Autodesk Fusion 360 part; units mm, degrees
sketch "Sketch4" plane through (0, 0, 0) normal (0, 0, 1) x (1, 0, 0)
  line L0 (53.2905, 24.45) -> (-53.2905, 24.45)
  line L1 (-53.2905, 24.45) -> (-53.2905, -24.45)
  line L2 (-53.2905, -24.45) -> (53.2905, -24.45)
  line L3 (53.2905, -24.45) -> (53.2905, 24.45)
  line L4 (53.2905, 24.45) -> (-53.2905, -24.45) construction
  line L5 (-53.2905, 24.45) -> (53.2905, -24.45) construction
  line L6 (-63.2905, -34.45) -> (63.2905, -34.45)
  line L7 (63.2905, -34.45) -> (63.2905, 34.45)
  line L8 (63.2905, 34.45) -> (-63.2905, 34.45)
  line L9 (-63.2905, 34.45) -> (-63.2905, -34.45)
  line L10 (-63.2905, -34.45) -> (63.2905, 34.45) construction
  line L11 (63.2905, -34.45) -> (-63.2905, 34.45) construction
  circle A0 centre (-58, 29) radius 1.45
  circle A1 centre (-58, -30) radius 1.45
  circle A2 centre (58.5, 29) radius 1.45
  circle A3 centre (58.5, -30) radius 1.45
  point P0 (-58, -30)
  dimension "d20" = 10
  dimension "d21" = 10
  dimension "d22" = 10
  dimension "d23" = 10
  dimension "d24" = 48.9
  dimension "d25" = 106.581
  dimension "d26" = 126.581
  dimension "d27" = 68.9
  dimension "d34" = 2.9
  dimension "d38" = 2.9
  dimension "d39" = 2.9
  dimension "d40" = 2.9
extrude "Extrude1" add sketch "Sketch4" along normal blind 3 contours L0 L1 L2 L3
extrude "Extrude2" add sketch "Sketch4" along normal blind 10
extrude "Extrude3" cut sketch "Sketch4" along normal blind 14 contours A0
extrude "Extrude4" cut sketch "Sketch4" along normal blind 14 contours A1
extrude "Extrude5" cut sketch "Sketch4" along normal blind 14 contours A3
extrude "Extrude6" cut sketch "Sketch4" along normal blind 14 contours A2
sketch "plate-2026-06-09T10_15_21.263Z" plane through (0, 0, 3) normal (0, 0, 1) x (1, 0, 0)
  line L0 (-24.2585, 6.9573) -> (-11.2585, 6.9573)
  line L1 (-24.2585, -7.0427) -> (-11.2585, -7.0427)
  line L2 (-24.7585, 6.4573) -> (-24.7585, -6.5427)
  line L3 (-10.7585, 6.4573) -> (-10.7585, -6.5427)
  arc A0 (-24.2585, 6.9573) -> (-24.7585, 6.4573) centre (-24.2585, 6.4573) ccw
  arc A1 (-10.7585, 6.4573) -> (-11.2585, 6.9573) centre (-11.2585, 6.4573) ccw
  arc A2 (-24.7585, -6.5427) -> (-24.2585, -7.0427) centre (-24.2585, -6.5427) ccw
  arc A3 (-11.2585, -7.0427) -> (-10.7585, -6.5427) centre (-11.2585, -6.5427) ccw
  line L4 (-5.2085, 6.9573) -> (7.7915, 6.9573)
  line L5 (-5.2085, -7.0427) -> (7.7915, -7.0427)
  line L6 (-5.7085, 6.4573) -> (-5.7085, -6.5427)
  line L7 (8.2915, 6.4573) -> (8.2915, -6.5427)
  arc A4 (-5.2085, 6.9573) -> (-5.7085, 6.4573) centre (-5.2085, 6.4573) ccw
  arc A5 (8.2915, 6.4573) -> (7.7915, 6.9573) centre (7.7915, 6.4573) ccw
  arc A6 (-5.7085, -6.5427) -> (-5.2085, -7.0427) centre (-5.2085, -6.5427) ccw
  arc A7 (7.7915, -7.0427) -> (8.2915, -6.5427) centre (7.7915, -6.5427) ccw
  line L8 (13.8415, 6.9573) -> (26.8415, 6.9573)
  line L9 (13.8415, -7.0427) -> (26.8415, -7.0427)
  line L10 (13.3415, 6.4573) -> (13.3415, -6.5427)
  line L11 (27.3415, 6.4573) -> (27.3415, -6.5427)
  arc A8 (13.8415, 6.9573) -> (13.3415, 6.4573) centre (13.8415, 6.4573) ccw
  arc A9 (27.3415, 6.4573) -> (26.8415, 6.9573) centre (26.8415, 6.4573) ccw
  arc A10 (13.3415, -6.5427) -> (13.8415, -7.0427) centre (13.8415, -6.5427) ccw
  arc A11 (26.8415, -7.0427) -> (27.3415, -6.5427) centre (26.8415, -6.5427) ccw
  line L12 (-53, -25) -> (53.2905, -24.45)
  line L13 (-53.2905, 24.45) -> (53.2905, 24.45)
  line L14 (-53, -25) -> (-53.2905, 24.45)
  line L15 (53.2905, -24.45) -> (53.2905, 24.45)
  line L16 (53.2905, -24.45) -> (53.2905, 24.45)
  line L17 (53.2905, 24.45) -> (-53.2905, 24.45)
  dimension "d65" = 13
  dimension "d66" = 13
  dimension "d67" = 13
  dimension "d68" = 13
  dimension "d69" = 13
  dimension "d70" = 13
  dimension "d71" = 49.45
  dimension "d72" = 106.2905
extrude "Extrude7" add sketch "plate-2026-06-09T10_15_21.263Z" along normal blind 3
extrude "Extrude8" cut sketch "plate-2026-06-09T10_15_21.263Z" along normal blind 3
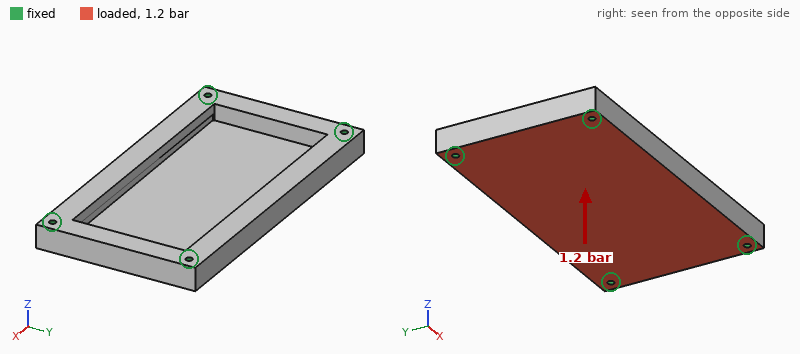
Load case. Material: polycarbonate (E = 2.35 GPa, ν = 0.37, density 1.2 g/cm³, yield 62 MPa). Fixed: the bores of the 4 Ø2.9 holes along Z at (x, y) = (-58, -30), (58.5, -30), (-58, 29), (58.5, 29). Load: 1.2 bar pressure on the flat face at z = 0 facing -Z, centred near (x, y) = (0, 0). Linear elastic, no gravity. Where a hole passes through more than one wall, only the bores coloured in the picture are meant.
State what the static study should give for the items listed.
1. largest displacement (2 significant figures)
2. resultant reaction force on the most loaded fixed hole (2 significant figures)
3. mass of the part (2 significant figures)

1.5 mm
310 N
60 g
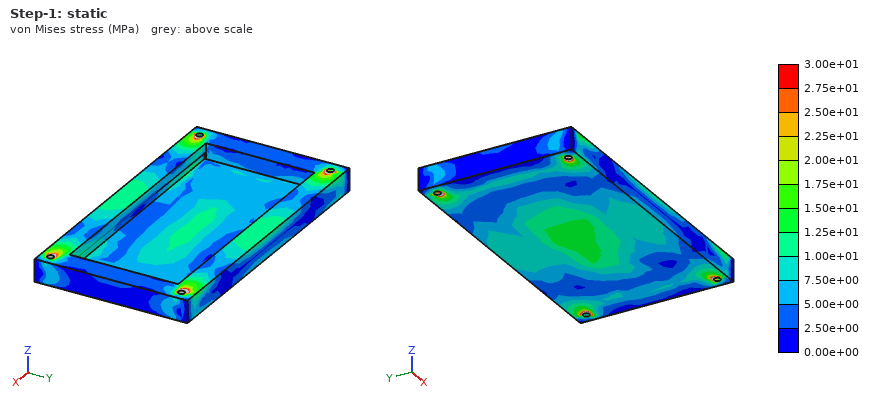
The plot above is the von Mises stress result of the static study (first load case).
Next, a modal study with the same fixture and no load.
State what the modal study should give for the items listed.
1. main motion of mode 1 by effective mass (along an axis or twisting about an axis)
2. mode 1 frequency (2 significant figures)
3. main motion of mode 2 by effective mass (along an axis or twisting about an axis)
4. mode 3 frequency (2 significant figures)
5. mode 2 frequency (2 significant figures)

along Z
800 Hz
twisting about X
1600 Hz
1000 Hz
